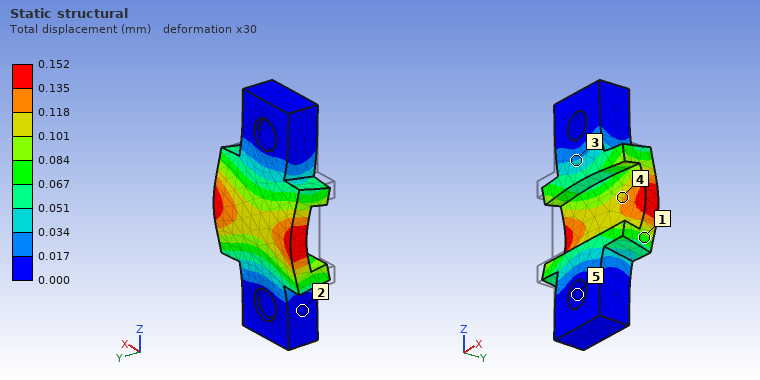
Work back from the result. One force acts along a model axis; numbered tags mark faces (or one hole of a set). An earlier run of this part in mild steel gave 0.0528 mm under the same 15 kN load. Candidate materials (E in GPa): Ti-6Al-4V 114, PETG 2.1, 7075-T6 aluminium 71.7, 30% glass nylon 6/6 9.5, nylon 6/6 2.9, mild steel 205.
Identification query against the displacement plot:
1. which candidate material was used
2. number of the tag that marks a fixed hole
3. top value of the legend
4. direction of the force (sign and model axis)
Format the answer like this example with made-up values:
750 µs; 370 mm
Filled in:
7075-T6 aluminium; 5; 0.152 mm; +Y
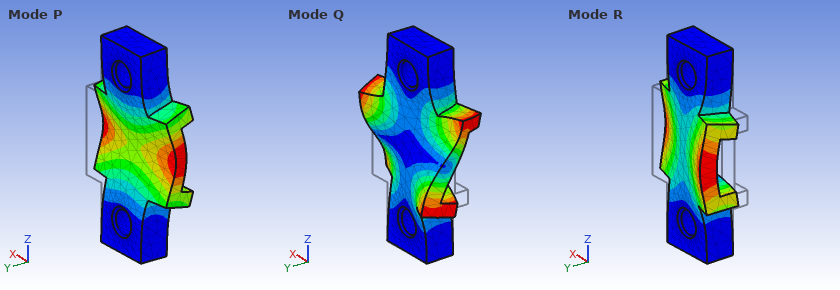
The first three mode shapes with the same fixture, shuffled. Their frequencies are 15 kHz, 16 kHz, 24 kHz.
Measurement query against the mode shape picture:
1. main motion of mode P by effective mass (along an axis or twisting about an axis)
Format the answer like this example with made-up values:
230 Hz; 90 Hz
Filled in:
along Y
